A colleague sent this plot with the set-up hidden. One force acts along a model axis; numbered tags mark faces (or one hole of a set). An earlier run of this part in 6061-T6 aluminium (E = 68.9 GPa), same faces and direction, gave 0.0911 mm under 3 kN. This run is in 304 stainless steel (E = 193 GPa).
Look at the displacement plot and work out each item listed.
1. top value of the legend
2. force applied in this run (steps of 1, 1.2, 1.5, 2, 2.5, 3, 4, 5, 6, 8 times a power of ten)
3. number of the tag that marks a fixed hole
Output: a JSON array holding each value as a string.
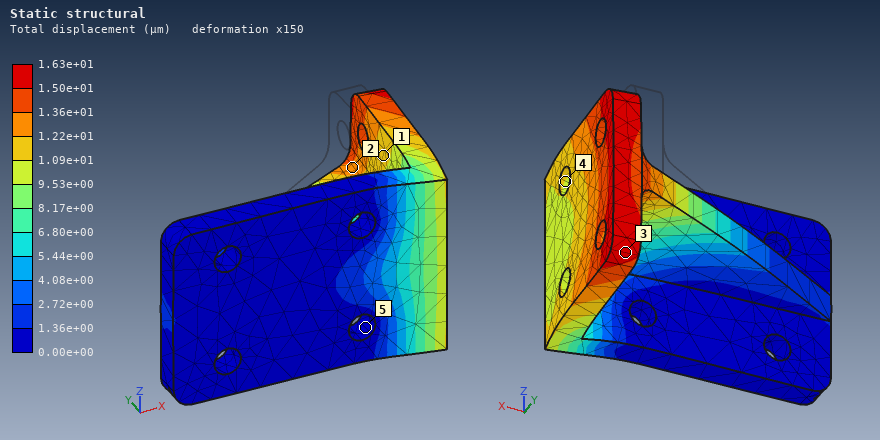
["1.63e+01 µm", "1.5 kN", "5"]
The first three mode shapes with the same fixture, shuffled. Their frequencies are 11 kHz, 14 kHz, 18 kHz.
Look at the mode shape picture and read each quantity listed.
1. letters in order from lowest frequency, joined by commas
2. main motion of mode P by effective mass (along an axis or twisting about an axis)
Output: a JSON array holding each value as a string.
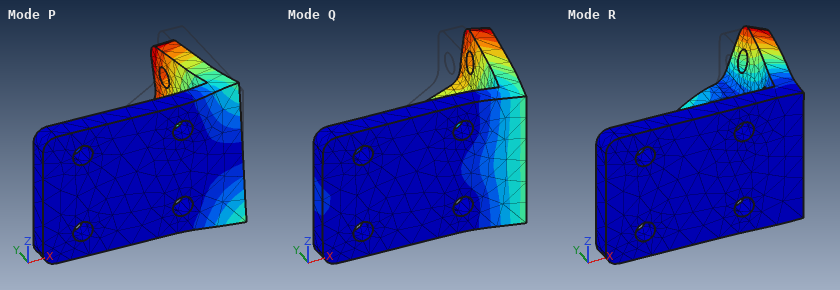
["P, Q, R", "along Z"]
